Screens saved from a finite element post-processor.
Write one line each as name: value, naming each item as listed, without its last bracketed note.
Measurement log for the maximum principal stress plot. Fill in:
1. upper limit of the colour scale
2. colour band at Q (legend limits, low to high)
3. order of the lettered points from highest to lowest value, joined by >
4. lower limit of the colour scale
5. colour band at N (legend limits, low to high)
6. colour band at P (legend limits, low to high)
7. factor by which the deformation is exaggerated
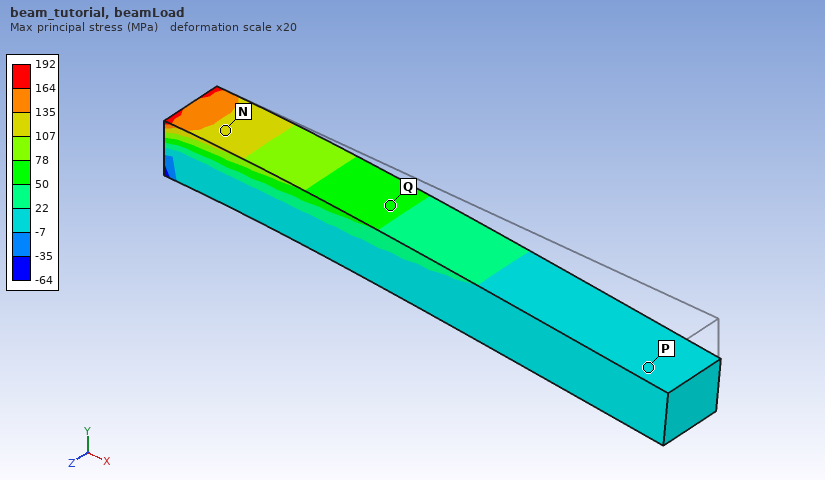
upper limit of the colour scale: 192 MPa
colour band at Q: 50 to 78 MPa
order of the lettered points from highest to lowest value, joined by >: N > Q > P
lower limit of the colour scale: -64 MPa
colour band at N: 107 to 135 MPa
colour band at P: -7 to 22 MPa
factor by which the deformation is exaggerated: 20
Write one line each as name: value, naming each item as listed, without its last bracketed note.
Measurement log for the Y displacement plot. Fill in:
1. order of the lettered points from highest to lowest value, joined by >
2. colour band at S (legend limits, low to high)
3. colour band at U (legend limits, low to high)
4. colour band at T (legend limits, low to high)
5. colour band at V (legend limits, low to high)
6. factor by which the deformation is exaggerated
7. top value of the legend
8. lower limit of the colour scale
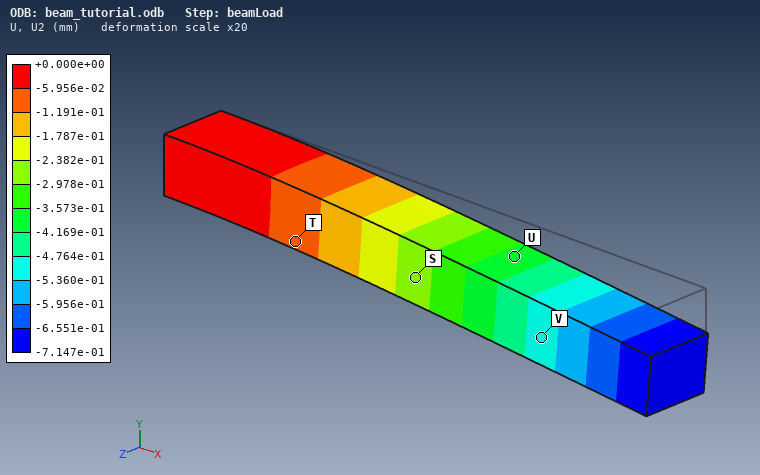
order of the lettered points from highest to lowest value, joined by >: T > S > U > V
colour band at S: -2.978e-01 to -2.382e-01 mm
colour band at U: -4.169e-01 to -3.573e-01 mm
colour band at T: -1.191e-01 to -5.956e-02 mm
colour band at V: -5.360e-01 to -4.764e-01 mm
factor by which the deformation is exaggerated: 20
top value of the legend: +0.000e+00 mm
lower limit of the colour scale: -7.147e-01 mm
